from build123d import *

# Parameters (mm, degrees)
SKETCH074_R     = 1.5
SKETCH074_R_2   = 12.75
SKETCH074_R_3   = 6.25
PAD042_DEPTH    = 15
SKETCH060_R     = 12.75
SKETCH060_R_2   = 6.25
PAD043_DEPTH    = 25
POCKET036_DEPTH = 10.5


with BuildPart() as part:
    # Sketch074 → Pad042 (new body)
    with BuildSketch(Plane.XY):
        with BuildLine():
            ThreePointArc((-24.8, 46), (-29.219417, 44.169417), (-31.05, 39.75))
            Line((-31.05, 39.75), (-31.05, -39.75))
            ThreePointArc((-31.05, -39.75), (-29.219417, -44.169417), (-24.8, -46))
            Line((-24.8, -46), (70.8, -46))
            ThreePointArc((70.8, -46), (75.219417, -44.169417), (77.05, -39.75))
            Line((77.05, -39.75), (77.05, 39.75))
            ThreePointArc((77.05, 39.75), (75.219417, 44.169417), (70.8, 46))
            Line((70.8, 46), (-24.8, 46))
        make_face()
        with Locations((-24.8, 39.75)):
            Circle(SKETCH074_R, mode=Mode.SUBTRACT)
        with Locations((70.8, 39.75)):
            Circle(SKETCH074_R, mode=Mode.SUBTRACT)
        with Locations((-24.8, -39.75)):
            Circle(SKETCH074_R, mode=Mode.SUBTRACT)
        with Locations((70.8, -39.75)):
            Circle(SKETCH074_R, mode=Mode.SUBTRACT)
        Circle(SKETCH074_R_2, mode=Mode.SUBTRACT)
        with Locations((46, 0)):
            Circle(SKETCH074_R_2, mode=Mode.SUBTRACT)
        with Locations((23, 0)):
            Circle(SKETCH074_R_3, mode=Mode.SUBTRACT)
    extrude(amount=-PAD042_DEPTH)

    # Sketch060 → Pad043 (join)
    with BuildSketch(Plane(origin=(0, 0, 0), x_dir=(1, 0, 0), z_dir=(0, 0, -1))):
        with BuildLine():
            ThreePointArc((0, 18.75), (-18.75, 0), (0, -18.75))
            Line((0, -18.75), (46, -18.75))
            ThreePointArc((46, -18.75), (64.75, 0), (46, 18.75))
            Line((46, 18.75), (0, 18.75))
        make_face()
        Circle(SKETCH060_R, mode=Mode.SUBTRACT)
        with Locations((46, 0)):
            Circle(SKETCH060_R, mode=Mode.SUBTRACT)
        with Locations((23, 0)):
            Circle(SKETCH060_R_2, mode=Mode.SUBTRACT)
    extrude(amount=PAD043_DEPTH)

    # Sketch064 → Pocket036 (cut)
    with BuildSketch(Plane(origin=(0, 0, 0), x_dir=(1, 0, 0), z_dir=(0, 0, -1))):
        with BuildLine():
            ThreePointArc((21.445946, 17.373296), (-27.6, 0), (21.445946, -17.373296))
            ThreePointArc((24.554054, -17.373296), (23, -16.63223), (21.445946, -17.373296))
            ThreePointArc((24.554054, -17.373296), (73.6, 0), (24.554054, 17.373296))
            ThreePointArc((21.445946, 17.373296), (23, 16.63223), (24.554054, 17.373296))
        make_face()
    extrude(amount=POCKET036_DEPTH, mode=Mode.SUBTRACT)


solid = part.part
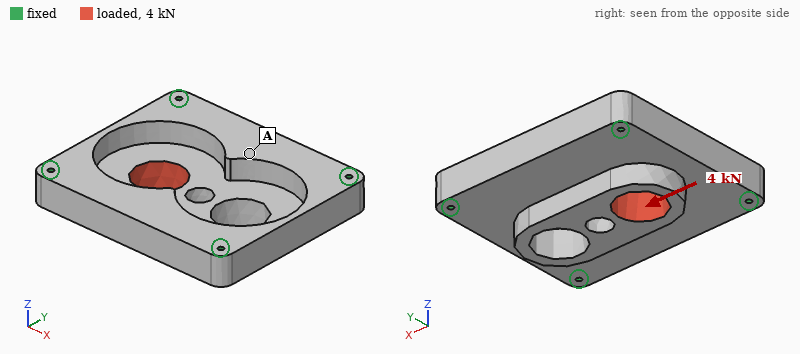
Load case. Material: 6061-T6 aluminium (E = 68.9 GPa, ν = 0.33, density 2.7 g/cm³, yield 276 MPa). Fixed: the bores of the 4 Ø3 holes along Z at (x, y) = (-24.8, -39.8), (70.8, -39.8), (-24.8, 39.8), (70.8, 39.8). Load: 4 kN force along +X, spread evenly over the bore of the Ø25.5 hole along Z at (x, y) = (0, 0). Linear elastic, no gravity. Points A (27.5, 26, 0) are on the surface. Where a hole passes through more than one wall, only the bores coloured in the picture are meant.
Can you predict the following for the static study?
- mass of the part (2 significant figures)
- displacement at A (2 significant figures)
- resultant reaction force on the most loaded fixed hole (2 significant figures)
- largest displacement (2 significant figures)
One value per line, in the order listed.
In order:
300 g
2.8 µm
1.1 kN
12 µm
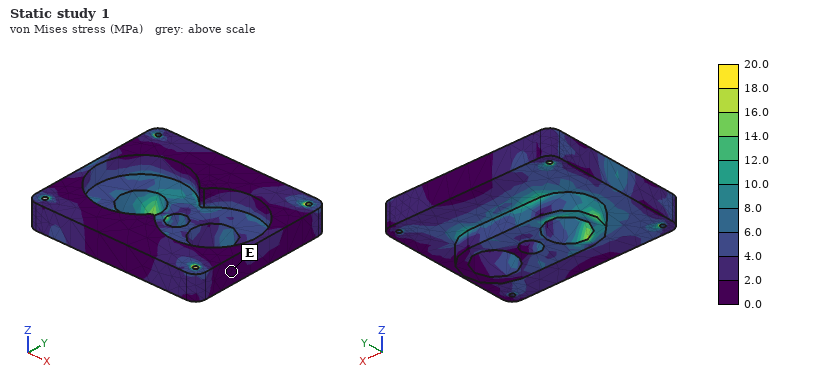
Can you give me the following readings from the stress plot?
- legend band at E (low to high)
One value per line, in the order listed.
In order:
0.0 to 2.0 MPa
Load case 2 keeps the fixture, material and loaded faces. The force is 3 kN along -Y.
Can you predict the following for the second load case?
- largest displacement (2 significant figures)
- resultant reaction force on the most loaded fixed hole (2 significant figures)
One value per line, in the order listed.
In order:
7.8 µm
1.2 kN
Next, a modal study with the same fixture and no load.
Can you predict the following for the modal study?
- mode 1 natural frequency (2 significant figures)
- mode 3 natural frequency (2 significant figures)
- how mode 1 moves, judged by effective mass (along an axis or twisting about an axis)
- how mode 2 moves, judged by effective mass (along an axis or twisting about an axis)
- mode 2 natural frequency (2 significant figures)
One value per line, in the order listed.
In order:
5300 Hz
8400 Hz
along Z
twisting about X
6400 Hz
